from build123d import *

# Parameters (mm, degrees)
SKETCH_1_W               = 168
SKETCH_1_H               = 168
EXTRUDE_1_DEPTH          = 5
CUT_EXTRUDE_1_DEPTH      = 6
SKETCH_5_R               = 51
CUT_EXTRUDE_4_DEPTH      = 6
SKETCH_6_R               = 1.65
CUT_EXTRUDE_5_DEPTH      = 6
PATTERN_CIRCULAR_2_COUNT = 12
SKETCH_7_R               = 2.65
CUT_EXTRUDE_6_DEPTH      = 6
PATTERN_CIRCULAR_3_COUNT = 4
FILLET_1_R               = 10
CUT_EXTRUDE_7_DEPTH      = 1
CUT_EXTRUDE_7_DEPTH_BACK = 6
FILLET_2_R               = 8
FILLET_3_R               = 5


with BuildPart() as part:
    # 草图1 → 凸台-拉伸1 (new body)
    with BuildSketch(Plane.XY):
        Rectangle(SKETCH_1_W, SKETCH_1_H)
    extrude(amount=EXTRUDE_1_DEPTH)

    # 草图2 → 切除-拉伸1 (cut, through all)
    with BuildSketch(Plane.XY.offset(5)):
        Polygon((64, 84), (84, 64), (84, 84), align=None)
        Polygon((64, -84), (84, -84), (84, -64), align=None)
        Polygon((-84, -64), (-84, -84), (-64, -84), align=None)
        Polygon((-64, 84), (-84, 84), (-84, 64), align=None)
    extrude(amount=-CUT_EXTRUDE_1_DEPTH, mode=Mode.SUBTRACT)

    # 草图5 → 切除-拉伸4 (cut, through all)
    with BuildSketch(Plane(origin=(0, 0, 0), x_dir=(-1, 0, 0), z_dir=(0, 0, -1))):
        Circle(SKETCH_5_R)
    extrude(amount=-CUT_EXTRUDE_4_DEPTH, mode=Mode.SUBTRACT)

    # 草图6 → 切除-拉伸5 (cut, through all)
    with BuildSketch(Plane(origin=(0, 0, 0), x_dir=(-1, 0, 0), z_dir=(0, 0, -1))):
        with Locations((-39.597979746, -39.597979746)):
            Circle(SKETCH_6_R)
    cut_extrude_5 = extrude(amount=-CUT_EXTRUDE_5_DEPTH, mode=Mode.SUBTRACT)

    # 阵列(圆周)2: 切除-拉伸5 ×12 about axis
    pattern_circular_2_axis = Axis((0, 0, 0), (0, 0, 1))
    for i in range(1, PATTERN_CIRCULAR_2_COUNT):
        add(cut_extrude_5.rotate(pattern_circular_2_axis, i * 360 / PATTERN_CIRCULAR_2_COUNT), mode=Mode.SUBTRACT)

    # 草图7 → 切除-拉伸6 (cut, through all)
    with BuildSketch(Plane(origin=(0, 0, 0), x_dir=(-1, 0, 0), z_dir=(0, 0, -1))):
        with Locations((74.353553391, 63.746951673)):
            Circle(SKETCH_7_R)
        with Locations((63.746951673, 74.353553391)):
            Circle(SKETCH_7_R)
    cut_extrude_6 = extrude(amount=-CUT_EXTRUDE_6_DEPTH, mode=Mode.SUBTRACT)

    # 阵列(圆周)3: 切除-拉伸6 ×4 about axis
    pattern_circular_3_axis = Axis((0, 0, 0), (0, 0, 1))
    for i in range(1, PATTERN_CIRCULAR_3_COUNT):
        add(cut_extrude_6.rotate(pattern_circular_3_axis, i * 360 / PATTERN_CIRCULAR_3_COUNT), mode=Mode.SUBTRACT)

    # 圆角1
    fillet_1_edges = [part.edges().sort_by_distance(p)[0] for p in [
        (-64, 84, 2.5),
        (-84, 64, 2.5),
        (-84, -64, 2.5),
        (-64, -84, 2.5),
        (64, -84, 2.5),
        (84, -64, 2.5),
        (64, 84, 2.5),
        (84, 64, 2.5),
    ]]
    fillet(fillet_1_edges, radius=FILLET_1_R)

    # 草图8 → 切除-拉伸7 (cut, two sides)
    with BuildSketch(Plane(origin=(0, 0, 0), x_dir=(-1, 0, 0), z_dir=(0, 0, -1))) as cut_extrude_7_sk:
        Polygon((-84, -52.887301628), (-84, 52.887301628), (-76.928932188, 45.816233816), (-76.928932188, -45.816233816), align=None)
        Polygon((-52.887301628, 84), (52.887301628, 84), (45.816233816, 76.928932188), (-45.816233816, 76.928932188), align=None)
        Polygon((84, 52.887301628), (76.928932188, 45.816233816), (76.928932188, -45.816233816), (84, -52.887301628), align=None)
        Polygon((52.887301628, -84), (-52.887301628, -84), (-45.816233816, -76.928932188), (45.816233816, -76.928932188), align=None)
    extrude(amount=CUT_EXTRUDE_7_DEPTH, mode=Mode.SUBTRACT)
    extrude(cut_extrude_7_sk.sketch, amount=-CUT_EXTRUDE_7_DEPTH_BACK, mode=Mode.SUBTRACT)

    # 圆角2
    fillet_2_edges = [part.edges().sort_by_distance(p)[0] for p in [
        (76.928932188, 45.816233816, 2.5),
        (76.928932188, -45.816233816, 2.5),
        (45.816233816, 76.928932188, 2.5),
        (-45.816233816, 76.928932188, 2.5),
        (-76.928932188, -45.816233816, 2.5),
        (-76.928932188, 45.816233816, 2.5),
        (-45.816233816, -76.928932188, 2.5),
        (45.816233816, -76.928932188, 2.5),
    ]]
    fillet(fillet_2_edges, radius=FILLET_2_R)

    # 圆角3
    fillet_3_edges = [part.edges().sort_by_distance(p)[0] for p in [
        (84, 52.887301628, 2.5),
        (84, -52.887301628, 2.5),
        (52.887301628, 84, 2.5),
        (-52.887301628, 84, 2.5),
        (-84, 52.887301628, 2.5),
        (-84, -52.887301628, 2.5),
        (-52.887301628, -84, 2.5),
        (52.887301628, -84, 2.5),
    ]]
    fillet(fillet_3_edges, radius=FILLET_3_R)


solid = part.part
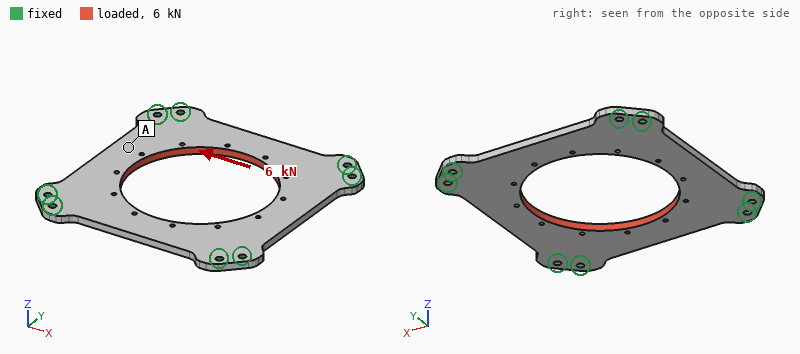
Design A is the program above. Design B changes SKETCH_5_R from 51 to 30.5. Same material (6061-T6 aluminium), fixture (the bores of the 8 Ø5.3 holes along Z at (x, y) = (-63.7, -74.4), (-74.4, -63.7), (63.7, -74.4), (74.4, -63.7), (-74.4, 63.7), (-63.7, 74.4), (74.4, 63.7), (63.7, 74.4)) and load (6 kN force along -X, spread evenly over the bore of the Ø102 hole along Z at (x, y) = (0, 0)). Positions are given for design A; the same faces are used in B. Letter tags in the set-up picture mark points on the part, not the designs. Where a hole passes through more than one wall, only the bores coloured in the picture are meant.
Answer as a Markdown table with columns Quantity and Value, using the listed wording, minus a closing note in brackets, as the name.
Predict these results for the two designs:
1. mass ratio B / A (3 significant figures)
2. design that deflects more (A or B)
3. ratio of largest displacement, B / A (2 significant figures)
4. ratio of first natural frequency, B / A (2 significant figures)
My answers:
| Quantity | Value |
|---|---|
| mass ratio B / A | 1.32 |
| design that deflects more | A |
| ratio of largest displacement, B / A | 0.63 |
| ratio of first natural frequency, B / A | 0.72 |
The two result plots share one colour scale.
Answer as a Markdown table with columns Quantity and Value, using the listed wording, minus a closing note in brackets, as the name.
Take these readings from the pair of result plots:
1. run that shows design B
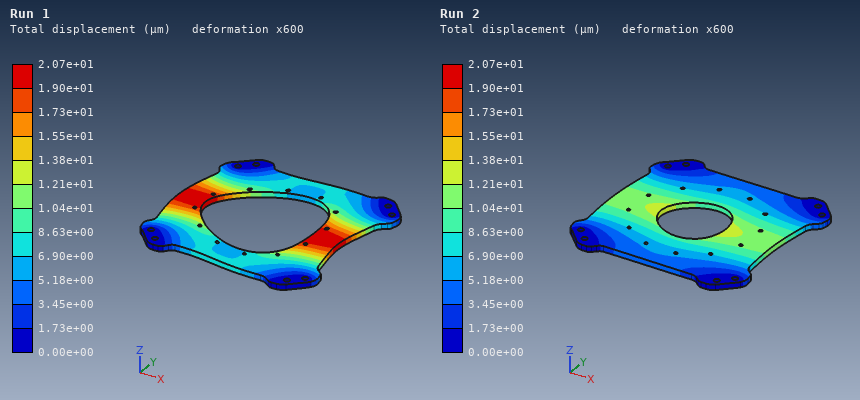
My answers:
| Quantity | Value |
|---|---|
| run that shows design B | Run 2 |
